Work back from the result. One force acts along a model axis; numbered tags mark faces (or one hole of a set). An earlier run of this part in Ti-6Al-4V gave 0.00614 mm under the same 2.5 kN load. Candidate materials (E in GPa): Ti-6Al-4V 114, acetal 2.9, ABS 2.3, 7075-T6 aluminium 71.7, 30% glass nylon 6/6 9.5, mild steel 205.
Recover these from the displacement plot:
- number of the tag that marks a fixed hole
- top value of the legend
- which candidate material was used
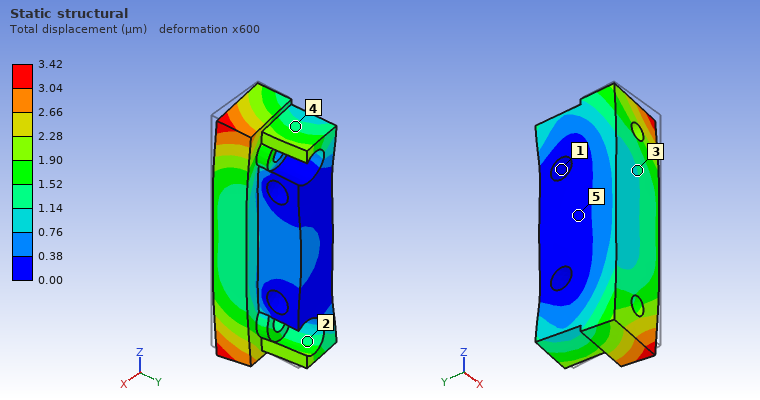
1
3.42 µm
mild steel
